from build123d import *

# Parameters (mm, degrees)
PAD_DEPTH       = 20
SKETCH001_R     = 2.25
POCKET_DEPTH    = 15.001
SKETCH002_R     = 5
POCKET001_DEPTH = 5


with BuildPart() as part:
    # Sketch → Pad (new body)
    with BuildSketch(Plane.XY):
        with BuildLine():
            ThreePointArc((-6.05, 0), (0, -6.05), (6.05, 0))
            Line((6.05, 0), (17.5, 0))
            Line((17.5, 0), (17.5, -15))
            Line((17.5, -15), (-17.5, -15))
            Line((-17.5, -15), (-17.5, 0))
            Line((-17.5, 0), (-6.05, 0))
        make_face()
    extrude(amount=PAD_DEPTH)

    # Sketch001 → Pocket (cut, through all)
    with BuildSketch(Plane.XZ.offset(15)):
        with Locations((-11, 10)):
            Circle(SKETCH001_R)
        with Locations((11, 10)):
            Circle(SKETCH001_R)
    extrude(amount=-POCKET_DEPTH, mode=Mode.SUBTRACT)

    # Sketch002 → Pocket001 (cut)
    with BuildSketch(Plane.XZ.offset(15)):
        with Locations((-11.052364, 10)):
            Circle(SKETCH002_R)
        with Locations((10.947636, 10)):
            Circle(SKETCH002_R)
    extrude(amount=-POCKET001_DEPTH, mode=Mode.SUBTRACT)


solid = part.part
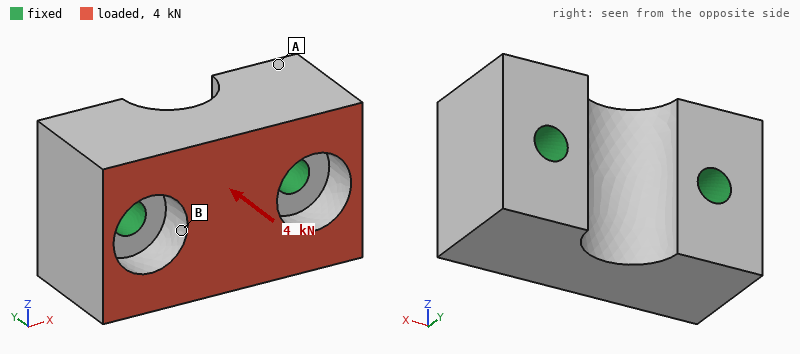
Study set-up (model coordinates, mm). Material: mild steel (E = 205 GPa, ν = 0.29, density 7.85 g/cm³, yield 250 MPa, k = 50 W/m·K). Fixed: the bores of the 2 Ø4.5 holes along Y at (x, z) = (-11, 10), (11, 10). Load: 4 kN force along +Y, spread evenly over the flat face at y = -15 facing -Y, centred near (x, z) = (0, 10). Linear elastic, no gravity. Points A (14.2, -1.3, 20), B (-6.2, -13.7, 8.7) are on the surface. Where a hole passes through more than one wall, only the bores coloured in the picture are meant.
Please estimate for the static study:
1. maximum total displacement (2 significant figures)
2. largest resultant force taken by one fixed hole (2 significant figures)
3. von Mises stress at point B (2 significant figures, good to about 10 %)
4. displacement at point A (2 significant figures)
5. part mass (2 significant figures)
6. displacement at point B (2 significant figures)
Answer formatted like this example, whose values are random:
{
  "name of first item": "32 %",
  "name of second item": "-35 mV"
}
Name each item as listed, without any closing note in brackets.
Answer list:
{
  "maximum total displacement": "1.4 µm",
  "largest resultant force taken by one fixed hole": "2.1 kN",
  "von Mises stress at point B": "14 MPa",
  "displacement at point A": "0.75 µm",
  "part mass": "65 g",
  "displacement at point B": "0.97 µm"
}
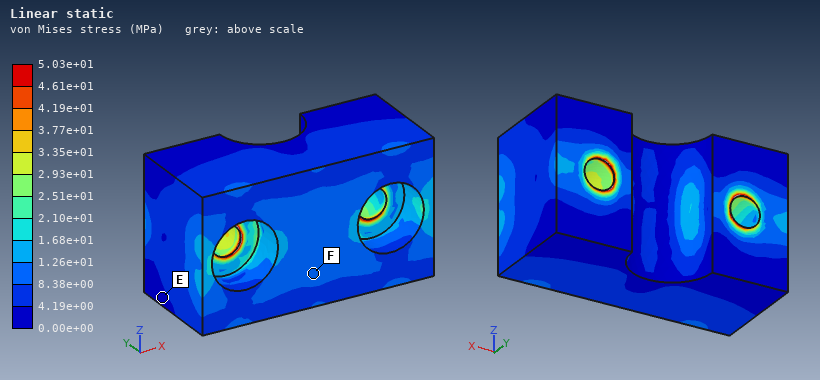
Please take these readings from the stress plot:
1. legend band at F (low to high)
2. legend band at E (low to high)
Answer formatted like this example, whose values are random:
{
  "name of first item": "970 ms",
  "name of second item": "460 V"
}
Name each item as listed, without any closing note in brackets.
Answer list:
{
  "legend band at F": "8.38e+00 to 1.26e+01 MPa",
  "legend band at E": "0.00e+00 to 4.19e+00 MPa"
}
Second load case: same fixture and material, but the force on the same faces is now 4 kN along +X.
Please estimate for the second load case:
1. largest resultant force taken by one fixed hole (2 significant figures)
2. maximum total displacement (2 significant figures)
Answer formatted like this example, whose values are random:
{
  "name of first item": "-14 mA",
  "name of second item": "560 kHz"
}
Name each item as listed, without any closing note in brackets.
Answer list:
{
  "largest resultant force taken by one fixed hole": "2.4 kN",
  "maximum total displacement": "3.2 µm"
}
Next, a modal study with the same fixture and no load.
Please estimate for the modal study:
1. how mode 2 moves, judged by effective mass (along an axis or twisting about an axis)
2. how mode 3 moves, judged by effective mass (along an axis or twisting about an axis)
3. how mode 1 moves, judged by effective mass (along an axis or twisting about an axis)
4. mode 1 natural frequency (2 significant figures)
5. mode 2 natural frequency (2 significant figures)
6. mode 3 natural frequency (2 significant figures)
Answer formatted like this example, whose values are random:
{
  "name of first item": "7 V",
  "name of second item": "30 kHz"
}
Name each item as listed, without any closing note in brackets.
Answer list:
{
  "how mode 2 moves, judged by effective mass": "twisting about Y",
  "how mode 3 moves, judged by effective mass": "along Y",
  "how mode 1 moves, judged by effective mass": "along Z",
  "mode 1 natural frequency": "31 kHz",
  "mode 2 natural frequency": "42 kHz",
  "mode 3 natural frequency": "47 kHz"
}
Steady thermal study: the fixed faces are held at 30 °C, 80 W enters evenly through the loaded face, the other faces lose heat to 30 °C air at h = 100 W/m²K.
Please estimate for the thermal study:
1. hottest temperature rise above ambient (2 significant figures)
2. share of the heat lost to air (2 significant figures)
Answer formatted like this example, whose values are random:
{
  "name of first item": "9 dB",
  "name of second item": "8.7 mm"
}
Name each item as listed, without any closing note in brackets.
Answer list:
{
  "hottest temperature rise above ambient": "42 K",
  "share of the heat lost to air": "6.3 %"
}
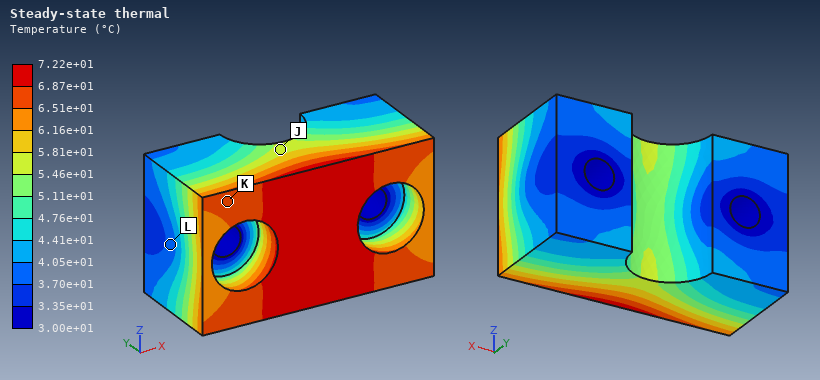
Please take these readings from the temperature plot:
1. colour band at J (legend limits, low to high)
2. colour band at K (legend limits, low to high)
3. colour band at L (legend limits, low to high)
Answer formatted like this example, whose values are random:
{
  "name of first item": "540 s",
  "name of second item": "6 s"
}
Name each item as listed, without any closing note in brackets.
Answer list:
{
  "colour band at J": "5.46e+01 to 5.81e+01 °C",
  "colour band at K": "6.51e+01 to 6.87e+01 °C",
  "colour band at L": "3.70e+01 to 4.05e+01 °C"
}
